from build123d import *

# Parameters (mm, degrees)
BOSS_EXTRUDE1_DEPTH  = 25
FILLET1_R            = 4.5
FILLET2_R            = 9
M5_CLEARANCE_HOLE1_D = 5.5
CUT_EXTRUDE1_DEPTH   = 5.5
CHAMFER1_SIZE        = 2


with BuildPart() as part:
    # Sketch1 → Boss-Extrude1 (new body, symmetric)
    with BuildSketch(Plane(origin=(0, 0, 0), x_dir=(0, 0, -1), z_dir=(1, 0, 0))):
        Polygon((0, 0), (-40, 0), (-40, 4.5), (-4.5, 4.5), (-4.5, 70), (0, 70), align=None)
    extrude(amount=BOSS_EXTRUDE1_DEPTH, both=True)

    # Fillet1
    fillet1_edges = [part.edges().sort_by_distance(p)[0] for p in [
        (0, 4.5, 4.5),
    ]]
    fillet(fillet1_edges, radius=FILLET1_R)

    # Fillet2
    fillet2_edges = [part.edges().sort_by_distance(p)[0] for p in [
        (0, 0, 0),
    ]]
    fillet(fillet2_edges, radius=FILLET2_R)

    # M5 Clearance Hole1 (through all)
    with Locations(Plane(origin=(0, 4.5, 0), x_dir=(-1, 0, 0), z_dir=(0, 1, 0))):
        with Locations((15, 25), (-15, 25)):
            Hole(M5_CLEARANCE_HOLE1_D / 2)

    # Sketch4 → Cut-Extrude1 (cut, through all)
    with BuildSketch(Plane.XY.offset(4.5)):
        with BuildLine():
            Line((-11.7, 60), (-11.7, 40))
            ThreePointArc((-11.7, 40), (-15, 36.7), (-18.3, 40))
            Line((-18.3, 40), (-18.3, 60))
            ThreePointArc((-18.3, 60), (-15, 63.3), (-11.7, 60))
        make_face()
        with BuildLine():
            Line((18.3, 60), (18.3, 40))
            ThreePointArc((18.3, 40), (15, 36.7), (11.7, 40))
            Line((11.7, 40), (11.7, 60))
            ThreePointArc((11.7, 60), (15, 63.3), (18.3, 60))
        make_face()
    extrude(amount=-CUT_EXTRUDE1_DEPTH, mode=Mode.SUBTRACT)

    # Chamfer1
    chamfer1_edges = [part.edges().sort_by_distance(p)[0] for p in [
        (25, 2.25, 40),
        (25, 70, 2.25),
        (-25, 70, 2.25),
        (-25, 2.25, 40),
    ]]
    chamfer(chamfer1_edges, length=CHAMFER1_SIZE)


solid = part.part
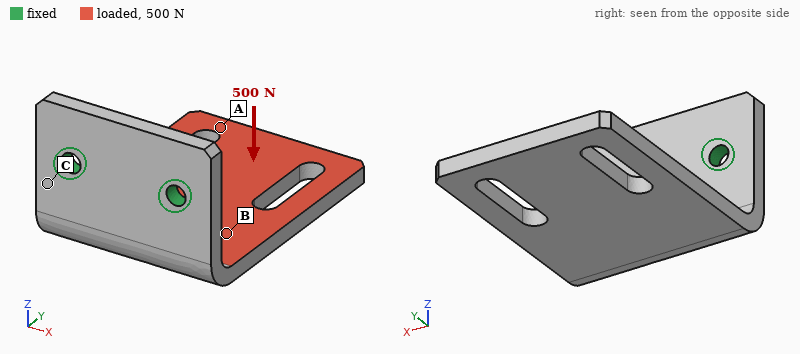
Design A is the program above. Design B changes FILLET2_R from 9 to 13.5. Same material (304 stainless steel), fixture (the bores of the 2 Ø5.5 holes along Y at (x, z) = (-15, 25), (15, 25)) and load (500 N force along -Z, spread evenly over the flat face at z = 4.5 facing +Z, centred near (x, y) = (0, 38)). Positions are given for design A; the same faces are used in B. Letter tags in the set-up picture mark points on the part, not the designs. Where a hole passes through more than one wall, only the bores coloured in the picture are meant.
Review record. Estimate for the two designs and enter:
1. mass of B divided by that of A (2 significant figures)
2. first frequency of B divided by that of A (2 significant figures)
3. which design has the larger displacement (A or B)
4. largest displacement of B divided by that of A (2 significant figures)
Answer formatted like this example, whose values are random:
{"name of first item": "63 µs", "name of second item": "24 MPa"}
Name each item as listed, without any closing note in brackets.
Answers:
{"mass of B divided by that of A": "0.95", "first frequency of B divided by that of A": "0.79", "which design has the larger displacement": "B", "largest displacement of B divided by that of A": "1.6"}
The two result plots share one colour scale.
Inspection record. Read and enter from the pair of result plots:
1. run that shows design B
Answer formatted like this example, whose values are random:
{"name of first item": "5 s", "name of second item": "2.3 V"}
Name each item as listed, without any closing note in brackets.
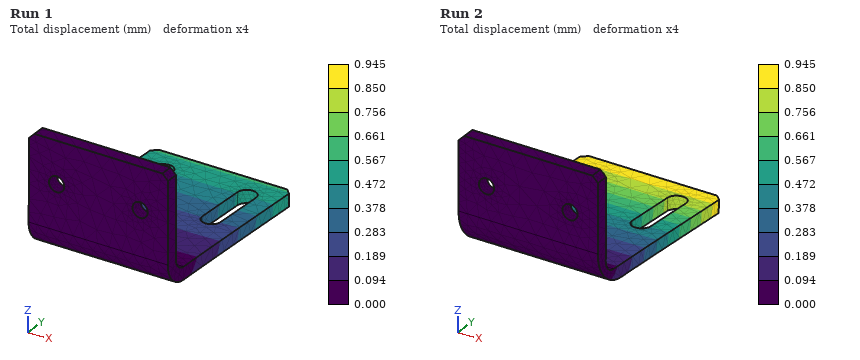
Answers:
{"run that shows design B": "Run 2"}
